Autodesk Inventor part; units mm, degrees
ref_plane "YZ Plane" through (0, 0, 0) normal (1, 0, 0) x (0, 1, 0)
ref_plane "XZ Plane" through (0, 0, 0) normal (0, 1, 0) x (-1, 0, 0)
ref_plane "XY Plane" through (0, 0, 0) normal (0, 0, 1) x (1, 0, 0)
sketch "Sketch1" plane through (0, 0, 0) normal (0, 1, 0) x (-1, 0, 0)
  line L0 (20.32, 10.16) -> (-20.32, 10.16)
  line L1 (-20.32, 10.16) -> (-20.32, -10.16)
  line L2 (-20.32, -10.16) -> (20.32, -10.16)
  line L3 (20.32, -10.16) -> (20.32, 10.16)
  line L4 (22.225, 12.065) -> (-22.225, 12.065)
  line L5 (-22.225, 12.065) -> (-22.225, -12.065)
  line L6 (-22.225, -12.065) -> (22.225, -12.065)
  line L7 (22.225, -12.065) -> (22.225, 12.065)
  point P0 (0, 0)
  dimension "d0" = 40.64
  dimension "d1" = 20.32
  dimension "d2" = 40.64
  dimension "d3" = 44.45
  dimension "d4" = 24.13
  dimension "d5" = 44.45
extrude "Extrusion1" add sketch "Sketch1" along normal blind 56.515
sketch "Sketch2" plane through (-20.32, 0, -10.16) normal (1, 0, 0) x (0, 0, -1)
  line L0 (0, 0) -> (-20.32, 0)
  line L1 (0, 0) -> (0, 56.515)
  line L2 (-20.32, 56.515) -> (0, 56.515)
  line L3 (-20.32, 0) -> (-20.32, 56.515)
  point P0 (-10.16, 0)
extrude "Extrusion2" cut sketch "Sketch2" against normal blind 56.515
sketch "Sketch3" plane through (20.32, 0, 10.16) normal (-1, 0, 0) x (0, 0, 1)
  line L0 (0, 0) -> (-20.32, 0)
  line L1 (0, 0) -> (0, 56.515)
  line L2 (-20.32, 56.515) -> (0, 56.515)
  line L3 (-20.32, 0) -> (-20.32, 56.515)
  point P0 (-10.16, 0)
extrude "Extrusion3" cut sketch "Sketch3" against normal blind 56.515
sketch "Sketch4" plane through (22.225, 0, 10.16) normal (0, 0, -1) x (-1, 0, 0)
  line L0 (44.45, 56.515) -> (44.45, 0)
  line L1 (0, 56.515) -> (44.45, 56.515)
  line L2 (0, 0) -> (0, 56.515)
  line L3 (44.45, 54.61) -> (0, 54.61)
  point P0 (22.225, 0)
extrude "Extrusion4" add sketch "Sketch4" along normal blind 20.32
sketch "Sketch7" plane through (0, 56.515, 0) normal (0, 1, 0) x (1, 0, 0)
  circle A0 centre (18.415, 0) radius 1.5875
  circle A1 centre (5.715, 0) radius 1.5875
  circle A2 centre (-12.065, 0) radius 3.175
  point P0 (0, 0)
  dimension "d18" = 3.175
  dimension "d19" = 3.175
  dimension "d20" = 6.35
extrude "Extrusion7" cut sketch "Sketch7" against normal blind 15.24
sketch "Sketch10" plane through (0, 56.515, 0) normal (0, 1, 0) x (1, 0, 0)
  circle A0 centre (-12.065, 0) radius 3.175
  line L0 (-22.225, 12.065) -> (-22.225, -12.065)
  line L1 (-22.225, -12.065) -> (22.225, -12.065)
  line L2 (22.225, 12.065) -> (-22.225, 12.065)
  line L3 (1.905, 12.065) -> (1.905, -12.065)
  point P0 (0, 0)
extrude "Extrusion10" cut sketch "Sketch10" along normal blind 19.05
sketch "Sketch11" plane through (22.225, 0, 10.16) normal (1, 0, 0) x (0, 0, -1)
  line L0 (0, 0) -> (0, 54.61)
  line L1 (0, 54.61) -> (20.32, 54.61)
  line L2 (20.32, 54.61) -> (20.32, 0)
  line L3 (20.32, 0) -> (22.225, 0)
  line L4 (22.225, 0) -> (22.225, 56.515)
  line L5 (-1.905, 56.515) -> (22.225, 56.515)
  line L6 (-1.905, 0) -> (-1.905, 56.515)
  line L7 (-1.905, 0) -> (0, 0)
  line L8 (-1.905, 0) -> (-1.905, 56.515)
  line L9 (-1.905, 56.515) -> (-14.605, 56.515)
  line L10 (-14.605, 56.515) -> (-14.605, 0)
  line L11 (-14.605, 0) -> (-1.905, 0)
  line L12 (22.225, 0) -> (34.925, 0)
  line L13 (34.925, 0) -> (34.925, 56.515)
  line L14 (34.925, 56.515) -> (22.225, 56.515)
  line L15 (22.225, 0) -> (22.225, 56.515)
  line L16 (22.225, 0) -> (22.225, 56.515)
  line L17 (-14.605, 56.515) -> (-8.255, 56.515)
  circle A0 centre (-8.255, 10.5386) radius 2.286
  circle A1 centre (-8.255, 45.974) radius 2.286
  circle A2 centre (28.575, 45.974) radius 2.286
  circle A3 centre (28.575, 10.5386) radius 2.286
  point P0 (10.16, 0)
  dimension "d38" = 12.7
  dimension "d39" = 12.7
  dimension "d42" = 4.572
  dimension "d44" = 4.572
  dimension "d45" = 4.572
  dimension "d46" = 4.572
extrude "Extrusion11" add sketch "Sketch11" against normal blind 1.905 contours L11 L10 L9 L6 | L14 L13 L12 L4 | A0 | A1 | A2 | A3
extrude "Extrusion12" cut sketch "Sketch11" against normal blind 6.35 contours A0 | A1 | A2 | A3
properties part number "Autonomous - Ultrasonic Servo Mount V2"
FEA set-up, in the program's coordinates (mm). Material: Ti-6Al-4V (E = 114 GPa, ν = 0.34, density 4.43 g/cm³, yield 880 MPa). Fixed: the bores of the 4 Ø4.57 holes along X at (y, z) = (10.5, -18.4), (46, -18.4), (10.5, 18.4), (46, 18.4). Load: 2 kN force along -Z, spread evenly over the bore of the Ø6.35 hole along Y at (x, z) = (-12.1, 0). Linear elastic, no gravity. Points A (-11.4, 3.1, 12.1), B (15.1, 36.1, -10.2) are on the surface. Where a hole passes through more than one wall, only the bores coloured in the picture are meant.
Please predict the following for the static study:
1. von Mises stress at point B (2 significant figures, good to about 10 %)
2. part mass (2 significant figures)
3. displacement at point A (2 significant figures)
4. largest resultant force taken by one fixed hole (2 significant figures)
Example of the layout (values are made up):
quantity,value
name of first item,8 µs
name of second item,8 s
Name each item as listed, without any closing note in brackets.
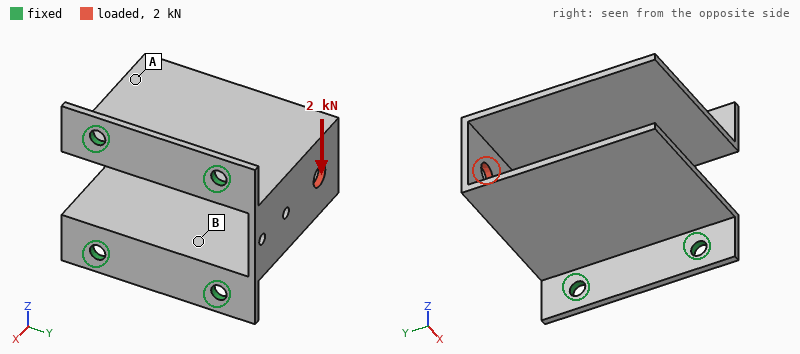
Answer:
quantity,value
von Mises stress at point B,120 MPa
part mass,61 g
displacement at point A,0.28 mm
largest resultant force taken by one fixed hole,2.8 kN
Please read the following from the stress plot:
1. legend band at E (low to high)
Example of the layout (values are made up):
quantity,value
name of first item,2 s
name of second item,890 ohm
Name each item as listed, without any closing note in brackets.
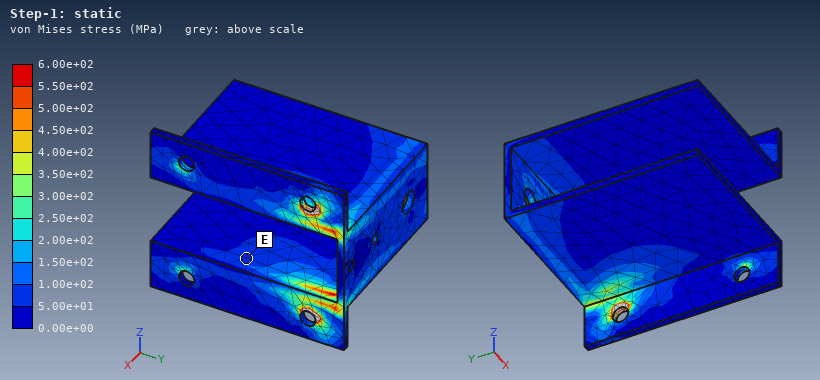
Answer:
quantity,value
legend band at E,5.00e+01 to 1.00e+02 MPa
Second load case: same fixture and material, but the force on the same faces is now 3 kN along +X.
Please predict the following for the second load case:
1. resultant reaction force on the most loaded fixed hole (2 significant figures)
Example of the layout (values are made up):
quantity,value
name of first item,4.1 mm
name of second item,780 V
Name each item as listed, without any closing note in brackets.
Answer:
quantity,value
resultant reaction force on the most loaded fixed hole,1.9 kN
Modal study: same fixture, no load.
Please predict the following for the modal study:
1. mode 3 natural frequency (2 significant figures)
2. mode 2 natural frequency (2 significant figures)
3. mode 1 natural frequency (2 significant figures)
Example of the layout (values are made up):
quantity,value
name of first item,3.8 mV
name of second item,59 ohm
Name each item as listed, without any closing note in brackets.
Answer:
quantity,value
mode 3 natural frequency,2900 Hz
mode 2 natural frequency,1100 Hz
mode 1 natural frequency,1100 Hz
